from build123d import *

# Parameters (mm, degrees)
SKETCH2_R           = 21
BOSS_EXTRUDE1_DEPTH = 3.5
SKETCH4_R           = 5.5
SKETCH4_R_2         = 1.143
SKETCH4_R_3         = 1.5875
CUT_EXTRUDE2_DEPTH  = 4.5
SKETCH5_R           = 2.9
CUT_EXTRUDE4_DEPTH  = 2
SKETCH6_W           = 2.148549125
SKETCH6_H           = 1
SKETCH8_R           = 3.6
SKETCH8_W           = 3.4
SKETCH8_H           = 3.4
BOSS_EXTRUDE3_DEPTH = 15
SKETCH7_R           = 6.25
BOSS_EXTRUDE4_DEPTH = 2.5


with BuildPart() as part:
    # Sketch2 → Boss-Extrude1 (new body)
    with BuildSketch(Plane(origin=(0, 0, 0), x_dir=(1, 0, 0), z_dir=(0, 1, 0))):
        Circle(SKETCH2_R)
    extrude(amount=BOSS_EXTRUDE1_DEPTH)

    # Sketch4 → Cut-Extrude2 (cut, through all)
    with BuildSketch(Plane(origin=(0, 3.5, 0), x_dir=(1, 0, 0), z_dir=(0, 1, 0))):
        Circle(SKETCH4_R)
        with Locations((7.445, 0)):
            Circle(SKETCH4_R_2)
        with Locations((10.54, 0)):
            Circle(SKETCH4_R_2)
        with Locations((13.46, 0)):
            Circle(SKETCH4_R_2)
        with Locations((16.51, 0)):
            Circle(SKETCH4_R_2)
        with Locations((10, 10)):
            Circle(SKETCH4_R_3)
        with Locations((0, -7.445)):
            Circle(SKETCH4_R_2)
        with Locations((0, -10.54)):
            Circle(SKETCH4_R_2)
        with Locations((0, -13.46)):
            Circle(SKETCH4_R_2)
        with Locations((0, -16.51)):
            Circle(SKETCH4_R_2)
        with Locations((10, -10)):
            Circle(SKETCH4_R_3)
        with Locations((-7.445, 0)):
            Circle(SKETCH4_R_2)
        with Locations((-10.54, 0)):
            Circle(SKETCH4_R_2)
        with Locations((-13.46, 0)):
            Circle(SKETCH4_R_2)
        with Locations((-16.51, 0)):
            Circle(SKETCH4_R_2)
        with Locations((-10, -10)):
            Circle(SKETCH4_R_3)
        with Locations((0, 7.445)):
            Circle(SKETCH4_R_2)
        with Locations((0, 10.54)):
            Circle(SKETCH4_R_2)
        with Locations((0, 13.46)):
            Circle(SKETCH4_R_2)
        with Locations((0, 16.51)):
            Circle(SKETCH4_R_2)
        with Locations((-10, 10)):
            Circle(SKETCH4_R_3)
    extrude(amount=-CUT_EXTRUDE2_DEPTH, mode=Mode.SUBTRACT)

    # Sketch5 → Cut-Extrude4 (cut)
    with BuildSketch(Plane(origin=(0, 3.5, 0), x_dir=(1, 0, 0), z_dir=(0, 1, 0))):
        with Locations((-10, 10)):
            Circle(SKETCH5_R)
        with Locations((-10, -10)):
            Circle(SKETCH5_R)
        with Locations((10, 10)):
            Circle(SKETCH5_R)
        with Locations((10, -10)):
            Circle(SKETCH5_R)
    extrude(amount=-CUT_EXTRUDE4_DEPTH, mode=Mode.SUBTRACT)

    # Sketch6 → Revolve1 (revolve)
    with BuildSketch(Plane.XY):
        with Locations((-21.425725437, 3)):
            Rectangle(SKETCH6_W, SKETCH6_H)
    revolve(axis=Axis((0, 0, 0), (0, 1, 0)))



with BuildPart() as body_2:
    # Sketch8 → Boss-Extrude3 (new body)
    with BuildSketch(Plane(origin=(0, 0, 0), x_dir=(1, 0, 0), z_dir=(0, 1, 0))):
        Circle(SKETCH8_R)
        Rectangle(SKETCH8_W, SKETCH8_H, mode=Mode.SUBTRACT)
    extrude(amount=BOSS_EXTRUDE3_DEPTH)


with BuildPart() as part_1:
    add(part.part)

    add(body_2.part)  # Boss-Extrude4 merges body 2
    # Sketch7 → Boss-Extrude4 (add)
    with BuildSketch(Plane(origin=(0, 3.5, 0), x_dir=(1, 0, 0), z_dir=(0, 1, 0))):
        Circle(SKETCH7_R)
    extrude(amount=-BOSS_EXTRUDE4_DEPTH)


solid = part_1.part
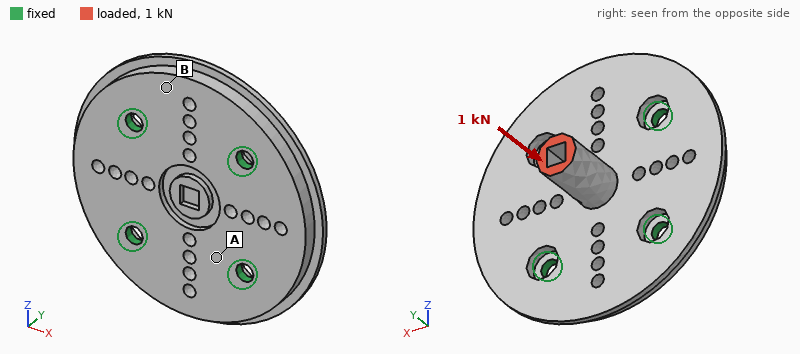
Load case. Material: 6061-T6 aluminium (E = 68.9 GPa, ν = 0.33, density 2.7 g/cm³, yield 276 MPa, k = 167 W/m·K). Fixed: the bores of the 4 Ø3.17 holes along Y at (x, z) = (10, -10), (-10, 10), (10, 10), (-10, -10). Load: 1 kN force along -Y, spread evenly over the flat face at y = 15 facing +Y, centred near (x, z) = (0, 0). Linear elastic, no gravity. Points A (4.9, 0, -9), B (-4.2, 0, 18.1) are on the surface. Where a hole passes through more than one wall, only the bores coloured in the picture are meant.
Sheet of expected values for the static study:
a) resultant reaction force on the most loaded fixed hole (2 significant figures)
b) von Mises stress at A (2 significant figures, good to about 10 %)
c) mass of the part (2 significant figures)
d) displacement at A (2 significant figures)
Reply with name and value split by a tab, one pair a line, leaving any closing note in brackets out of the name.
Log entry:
resultant reaction force on the most loaded fixed hole	500 N
von Mises stress at A	29 MPa
mass of the part	13 g
displacement at A	8.3 µm
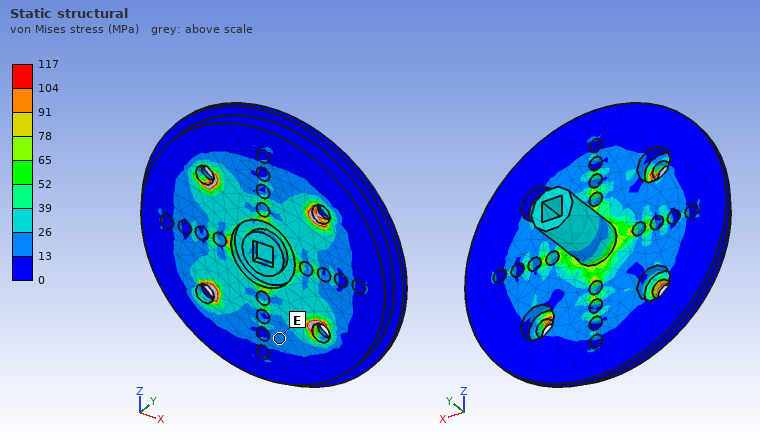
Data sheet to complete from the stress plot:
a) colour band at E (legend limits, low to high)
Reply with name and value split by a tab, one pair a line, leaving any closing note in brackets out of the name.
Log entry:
colour band at E	13 to 26 MPa
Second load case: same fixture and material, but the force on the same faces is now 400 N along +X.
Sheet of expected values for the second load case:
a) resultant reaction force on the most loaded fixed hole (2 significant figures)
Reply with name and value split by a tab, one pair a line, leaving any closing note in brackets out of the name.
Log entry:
resultant reaction force on the most loaded fixed hole	240 N
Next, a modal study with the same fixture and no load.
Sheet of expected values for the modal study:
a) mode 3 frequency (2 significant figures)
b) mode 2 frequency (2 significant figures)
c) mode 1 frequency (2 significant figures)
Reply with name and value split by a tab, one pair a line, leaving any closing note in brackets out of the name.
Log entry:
mode 3 frequency	16 kHz
mode 2 frequency	16 kHz
mode 1 frequency	14 kHz
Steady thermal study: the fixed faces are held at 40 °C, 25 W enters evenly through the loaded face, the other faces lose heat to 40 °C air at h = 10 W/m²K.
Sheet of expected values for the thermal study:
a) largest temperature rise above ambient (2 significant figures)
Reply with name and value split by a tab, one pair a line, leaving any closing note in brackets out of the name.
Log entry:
largest temperature rise above ambient	77 K
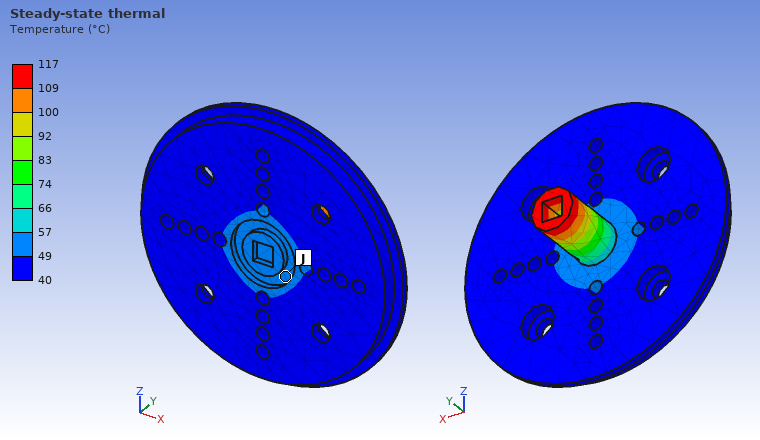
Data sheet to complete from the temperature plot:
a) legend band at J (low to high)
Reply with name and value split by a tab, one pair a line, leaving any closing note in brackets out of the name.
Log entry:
legend band at J	49 to 57 °C
